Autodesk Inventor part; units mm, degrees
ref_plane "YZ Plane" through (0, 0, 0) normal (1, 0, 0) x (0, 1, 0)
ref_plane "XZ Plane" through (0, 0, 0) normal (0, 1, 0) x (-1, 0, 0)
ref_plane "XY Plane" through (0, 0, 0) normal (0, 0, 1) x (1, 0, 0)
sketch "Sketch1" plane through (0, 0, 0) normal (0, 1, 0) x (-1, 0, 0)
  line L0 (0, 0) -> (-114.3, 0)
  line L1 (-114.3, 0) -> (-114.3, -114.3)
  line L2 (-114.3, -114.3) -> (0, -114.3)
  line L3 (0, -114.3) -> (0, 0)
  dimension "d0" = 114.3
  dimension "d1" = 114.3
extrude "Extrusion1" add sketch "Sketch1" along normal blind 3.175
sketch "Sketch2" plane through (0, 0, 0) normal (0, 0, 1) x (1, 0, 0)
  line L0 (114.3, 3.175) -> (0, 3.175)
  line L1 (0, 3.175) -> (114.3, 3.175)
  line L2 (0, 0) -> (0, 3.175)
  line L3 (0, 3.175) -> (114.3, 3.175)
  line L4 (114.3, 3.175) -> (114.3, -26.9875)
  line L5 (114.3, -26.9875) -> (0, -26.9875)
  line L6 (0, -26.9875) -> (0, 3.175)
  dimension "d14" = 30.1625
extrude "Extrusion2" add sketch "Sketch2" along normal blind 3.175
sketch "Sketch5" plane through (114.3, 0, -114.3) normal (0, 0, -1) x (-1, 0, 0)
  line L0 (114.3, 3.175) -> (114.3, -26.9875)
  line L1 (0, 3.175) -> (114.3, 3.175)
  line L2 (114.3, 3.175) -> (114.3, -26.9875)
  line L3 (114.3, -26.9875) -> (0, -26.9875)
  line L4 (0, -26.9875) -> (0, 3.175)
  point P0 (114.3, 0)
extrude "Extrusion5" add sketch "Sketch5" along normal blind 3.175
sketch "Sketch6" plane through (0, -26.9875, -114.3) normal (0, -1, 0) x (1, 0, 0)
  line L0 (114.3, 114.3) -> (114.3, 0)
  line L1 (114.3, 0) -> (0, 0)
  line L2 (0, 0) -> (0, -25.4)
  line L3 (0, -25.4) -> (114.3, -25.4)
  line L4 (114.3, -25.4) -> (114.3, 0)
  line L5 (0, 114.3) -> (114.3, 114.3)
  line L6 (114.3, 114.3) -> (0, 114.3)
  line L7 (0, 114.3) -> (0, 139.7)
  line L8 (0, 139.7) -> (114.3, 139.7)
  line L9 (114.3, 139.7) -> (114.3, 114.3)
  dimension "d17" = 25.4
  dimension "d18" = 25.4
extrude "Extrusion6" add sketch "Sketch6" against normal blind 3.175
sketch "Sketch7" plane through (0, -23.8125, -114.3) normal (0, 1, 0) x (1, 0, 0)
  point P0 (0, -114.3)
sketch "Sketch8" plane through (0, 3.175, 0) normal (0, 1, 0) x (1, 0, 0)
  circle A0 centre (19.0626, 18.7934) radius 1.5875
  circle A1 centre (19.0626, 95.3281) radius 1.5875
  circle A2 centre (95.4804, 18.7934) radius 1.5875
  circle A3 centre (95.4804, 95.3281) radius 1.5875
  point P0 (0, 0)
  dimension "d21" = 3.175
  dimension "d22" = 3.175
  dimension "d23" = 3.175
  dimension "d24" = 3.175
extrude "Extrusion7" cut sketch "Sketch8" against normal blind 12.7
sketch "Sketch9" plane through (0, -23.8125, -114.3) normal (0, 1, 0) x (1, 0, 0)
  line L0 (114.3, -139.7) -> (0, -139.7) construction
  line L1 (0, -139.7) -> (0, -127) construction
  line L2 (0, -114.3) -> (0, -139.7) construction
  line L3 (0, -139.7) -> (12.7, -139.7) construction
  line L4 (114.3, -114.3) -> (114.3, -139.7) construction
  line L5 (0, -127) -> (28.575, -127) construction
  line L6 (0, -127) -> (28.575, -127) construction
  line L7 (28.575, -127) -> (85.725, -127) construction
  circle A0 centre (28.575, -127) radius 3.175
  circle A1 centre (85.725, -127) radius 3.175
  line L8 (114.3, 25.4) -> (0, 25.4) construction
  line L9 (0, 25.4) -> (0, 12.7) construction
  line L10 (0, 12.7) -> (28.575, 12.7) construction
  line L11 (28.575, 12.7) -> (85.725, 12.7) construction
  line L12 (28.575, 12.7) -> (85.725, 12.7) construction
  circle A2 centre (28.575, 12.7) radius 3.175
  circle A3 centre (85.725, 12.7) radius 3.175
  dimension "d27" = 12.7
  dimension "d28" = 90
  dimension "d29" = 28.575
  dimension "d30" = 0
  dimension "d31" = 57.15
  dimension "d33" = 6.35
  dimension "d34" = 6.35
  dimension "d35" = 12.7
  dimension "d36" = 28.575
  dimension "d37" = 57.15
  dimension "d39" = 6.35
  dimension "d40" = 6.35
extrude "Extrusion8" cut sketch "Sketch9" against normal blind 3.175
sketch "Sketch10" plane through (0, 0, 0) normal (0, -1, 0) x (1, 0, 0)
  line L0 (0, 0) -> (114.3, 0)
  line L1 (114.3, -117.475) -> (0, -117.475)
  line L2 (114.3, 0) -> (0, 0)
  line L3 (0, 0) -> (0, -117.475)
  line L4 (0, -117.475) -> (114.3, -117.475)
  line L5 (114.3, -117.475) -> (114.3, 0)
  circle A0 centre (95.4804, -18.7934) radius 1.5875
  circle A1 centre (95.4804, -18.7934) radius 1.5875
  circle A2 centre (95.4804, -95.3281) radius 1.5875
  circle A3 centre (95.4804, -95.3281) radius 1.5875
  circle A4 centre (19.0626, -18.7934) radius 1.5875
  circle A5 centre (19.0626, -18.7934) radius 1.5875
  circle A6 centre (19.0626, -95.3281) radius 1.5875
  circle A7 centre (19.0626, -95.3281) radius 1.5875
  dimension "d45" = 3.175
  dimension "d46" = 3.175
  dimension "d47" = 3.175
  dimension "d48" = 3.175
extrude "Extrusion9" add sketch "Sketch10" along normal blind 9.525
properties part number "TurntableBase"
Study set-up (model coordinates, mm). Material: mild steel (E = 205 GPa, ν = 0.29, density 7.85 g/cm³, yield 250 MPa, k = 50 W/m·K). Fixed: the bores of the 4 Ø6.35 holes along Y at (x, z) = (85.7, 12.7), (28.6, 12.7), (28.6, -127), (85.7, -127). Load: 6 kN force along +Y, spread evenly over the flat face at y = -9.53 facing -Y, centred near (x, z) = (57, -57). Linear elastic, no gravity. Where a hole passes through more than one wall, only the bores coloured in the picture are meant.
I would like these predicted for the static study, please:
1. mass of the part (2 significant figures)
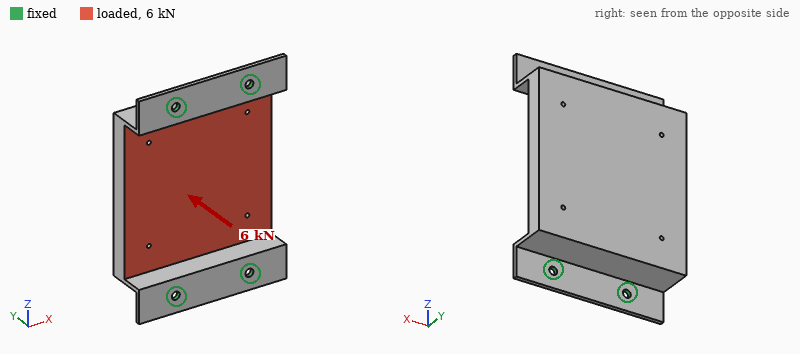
1.6 kg
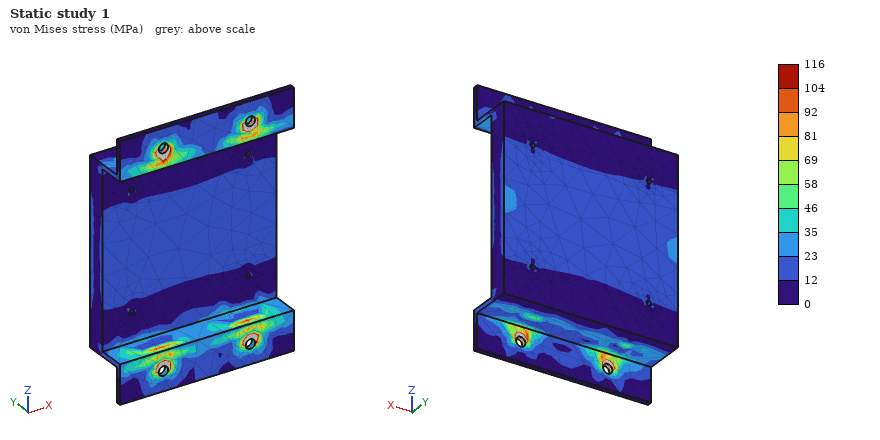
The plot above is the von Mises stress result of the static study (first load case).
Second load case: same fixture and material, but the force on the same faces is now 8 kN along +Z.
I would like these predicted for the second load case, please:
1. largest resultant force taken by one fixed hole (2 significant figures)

2.0 kN
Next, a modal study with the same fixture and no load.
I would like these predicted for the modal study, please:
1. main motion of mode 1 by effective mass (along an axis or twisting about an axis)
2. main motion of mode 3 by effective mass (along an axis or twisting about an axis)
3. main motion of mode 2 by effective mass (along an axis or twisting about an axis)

along Z
along Y
along X
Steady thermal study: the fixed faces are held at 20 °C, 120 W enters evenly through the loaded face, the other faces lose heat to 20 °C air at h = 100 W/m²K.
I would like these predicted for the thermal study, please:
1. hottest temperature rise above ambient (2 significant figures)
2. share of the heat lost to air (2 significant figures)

44 K
82 %
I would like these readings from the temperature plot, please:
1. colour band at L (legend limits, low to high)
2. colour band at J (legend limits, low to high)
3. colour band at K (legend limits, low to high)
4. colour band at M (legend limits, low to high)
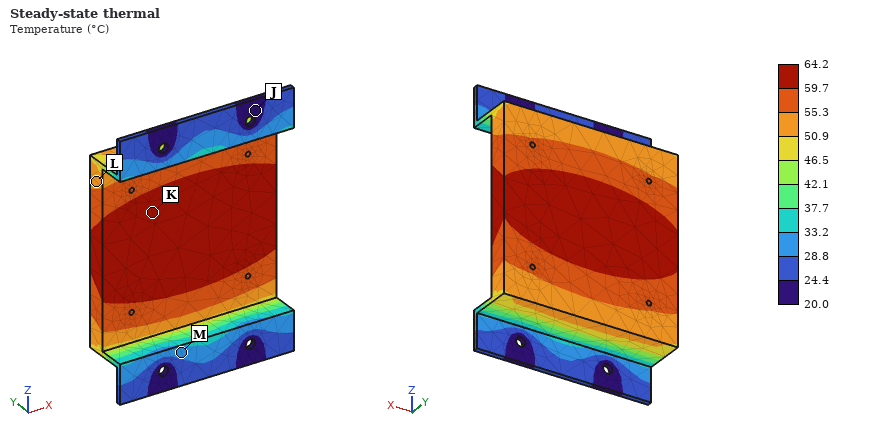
50.9 to 55.3 °C
20.0 to 24.4 °C
59.7 to 64.2 °C
28.8 to 33.2 °C
